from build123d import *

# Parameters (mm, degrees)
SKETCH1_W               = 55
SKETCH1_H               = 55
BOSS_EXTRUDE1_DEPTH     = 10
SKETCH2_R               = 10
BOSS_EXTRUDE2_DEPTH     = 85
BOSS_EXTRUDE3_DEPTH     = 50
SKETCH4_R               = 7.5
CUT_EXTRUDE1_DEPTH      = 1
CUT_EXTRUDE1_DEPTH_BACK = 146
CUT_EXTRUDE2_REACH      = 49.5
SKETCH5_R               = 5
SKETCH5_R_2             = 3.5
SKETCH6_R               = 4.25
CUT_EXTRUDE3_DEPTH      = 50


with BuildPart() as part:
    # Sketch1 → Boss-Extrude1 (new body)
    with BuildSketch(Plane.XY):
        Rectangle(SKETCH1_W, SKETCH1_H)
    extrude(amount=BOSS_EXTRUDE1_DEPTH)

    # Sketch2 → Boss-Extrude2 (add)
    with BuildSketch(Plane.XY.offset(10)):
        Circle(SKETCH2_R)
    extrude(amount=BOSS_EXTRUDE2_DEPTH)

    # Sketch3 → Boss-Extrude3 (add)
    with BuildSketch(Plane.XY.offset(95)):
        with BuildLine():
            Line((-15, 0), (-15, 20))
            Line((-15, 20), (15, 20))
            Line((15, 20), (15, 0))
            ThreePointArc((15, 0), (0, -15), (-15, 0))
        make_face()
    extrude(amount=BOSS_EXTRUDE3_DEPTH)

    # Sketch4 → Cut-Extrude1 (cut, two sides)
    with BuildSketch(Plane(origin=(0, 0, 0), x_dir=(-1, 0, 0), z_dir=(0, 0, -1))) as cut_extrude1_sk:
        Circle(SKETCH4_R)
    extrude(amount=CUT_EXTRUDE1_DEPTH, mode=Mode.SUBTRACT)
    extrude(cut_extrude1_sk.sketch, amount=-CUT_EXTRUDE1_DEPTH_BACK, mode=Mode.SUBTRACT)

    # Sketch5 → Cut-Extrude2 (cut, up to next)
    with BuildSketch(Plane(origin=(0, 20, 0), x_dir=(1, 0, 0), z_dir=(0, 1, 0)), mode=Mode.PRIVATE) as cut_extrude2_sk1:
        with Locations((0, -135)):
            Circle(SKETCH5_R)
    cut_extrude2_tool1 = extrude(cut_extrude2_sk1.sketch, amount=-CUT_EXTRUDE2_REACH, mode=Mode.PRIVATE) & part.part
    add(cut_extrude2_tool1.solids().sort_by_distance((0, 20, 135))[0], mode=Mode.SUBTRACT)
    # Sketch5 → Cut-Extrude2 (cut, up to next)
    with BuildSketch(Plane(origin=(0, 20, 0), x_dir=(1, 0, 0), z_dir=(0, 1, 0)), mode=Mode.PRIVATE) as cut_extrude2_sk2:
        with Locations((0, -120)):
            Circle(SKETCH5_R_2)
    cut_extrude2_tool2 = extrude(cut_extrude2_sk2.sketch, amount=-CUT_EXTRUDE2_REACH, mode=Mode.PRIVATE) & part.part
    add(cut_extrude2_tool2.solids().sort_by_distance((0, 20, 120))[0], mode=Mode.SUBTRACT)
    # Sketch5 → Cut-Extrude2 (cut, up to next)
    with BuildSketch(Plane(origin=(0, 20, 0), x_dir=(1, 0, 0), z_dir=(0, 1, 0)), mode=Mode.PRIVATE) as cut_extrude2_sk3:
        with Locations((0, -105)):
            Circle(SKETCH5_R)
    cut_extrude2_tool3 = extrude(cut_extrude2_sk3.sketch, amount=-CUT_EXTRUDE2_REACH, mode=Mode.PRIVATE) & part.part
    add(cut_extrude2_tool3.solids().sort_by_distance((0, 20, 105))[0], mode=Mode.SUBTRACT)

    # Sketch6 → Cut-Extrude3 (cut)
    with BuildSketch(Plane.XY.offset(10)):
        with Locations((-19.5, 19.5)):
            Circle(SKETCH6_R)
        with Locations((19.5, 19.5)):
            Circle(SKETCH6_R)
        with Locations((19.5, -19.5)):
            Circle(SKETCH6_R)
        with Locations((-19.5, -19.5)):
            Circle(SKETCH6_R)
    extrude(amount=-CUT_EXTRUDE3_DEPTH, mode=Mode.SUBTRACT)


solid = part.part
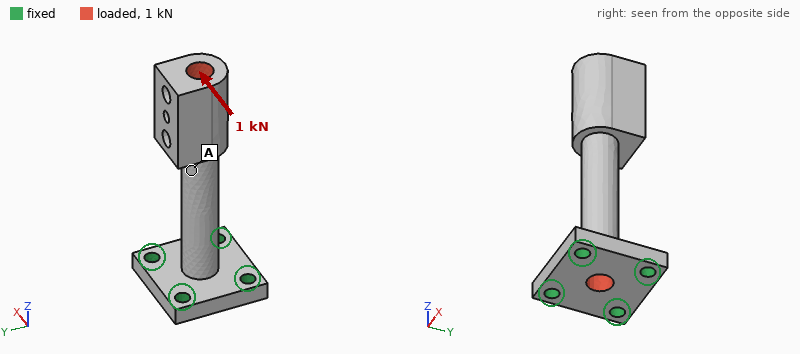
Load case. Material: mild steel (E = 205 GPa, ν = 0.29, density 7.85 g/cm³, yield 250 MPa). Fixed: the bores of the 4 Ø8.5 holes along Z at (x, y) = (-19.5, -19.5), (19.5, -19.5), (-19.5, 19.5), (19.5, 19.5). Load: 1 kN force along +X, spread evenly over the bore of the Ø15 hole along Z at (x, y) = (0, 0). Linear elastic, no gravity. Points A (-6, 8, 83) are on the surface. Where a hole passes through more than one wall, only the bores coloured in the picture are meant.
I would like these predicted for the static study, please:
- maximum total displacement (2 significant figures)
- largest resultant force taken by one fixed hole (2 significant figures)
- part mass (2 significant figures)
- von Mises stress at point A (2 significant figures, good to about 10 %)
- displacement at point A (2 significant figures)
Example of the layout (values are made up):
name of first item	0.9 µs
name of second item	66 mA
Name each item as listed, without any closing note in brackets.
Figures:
maximum total displacement	0.33 mm
largest resultant force taken by one fixed hole	1.1 kN
part mass	580 g
von Mises stress at point A	15 MPa
displacement at point A	0.15 mm
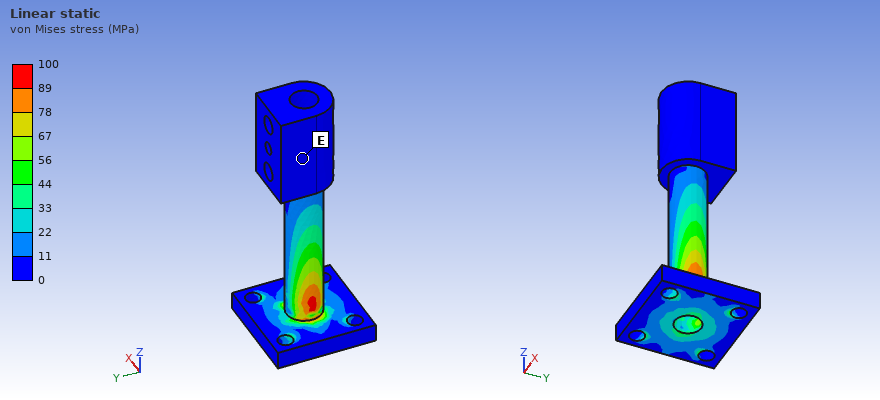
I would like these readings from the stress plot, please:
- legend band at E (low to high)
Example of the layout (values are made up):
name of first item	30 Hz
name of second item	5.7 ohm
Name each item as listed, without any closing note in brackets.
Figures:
legend band at E	0 to 11 MPa
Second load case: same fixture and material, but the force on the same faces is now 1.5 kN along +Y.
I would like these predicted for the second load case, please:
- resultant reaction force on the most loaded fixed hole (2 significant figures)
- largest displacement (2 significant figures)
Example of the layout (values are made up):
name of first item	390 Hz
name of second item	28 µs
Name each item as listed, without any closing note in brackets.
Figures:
resultant reaction force on the most loaded fixed hole	1.7 kN
largest displacement	0.49 mm
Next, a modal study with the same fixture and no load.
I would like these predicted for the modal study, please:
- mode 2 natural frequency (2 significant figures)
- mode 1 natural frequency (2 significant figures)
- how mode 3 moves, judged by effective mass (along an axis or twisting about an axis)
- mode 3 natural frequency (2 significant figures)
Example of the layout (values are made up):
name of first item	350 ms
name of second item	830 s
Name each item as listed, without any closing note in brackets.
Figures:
mode 2 natural frequency	400 Hz
mode 1 natural frequency	400 Hz
how mode 3 moves, judged by effective mass	twisting about Z
mode 3 natural frequency	2100 Hz
